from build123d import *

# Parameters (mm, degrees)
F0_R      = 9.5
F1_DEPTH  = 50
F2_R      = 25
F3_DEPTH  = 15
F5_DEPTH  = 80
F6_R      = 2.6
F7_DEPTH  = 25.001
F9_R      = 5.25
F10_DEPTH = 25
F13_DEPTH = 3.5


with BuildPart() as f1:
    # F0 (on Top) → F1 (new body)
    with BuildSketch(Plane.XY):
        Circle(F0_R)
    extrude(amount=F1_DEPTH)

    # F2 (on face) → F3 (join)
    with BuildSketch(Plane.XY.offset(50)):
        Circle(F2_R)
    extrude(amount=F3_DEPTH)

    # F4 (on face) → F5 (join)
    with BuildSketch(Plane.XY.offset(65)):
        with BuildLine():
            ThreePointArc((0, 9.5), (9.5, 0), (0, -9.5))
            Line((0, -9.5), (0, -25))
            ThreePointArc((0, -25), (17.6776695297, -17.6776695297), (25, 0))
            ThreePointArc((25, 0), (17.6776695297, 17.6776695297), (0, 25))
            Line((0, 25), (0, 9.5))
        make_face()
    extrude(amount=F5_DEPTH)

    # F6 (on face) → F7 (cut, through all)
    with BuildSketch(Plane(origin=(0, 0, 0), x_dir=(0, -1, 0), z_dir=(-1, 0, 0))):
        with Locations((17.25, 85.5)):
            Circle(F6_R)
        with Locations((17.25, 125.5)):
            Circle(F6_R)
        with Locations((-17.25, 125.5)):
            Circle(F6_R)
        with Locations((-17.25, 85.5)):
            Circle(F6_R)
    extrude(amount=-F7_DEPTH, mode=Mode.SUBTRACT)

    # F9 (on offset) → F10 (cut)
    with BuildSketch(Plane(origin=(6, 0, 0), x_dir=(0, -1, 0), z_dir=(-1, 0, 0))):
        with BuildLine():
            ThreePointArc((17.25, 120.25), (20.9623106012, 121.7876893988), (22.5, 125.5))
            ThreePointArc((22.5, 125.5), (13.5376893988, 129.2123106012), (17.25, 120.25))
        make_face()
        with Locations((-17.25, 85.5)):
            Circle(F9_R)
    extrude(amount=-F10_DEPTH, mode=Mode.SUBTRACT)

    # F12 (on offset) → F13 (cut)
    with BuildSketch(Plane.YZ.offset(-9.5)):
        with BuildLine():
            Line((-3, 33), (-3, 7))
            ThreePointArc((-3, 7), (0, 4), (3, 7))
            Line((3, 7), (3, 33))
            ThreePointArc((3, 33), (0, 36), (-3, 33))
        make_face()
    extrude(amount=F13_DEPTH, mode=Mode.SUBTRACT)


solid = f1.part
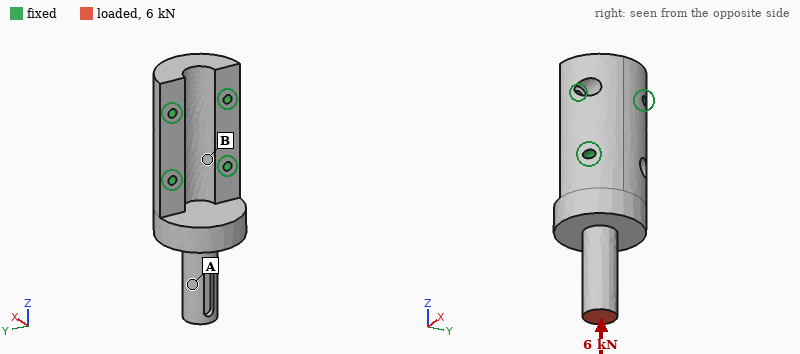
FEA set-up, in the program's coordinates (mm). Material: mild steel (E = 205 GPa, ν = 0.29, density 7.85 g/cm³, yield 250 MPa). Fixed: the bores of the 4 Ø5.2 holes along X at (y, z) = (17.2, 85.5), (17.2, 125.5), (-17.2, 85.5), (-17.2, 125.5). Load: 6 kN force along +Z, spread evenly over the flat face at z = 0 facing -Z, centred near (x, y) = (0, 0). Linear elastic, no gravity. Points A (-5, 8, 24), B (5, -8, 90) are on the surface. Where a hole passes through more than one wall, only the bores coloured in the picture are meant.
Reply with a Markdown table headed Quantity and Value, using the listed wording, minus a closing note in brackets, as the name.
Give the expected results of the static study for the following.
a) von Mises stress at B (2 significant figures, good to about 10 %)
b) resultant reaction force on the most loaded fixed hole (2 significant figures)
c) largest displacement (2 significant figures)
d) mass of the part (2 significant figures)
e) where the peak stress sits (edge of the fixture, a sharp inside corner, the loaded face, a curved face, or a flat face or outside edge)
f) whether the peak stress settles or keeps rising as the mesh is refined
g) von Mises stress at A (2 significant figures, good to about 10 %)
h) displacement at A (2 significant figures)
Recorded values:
| Quantity | Value |
|---|---|
| von Mises stress at B | 6.9 MPa |
| resultant reaction force on the most loaded fixed hole | 3.1 kN |
| largest displacement | 34 µm |
| mass of the part | 840 g |
| where the peak stress sits | edge of the fixture |
| whether the peak stress settles or keeps rising as the mesh is refined | keeps rising |
| von Mises stress at A | 27 MPa |
| displacement at A | 22 µm |
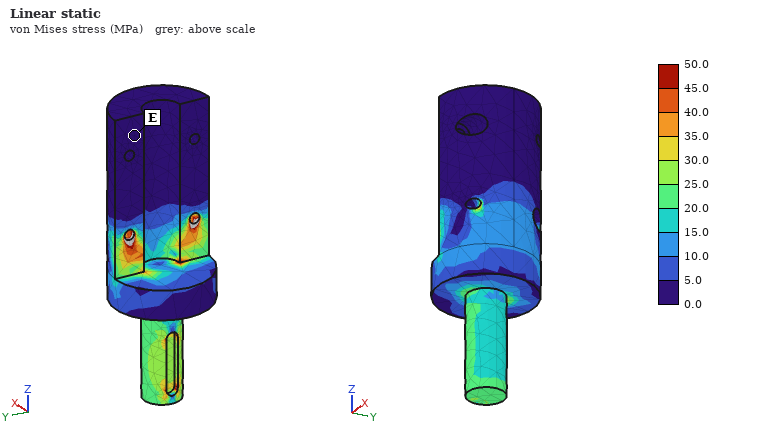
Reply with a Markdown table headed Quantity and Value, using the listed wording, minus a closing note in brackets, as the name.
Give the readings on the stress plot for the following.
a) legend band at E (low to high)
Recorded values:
| Quantity | Value |
|---|---|
| legend band at E | 0.0 to 5.0 MPa |
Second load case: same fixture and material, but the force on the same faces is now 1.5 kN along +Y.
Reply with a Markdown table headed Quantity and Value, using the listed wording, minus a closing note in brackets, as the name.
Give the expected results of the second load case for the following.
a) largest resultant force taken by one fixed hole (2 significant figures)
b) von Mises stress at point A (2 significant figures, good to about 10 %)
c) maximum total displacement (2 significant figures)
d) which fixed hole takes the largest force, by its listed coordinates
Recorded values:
| Quantity | Value |
|---|---|
| largest resultant force taken by one fixed hole | 3.6 kN |
| von Mises stress at point A | 44 MPa |
| maximum total displacement | 78 µm |
| which fixed hole takes the largest force, by its listed coordinates | (-17.2, 85.5) |
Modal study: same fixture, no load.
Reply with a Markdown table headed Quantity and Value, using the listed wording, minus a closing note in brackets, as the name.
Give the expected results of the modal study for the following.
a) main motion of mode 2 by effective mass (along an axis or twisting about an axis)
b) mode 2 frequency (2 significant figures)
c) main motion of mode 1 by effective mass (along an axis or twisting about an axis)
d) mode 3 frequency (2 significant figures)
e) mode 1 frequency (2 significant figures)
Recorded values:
| Quantity | Value |
|---|---|
| main motion of mode 2 by effective mass | along Y |
| mode 2 frequency | 3800 Hz |
| main motion of mode 1 by effective mass | along X |
| mode 3 frequency | 6400 Hz |
| mode 1 frequency | 2600 Hz |
